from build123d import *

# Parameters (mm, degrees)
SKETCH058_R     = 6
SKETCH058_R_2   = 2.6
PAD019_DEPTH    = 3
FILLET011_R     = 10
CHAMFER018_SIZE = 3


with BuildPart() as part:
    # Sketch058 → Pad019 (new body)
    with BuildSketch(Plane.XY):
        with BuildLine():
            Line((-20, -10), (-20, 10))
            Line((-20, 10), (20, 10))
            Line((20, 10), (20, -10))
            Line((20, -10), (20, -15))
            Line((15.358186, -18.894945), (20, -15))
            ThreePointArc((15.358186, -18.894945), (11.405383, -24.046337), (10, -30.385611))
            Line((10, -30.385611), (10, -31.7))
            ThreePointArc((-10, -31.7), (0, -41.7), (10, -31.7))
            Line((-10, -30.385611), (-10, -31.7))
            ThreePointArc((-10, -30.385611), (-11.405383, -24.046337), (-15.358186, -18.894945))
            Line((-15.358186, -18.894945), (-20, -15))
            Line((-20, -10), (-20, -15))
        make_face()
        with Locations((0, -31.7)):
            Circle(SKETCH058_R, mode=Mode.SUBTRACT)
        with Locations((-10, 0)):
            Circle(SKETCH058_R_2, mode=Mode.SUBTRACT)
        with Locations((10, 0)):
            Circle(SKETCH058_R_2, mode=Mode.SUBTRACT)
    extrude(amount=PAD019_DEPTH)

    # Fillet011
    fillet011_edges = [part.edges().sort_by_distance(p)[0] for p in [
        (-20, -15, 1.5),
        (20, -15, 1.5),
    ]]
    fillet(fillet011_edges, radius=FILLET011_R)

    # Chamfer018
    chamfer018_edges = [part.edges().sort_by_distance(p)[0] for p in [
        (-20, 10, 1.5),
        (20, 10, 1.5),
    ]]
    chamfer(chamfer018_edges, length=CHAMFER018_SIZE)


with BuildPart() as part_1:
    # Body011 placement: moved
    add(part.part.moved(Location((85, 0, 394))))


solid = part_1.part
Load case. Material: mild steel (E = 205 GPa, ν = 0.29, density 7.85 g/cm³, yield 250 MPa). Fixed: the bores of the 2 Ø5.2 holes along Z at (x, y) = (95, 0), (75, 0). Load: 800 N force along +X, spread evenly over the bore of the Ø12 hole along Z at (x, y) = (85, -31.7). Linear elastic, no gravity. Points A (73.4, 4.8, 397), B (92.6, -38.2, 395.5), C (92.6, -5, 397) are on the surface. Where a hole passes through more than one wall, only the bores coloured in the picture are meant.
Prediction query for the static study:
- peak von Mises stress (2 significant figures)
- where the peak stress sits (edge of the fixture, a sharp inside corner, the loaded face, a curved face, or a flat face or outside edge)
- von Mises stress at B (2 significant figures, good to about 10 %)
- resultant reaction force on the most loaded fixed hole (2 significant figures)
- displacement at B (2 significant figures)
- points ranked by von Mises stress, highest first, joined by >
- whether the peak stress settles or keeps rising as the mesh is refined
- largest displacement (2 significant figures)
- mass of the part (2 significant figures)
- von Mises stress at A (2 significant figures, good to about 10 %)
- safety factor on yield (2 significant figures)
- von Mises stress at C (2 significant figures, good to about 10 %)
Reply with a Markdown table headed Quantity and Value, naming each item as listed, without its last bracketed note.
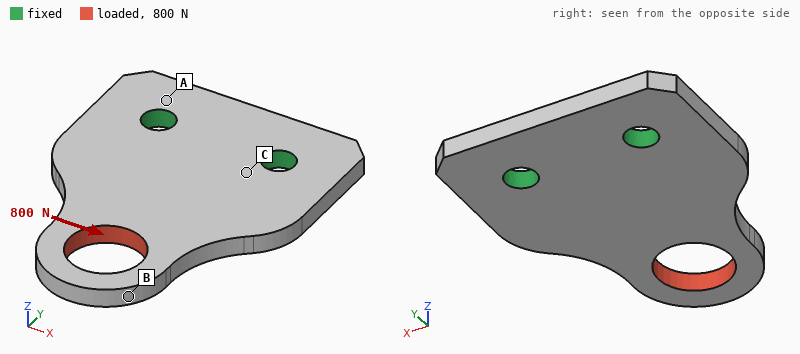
| Quantity | Value |
|---|---|
| peak von Mises stress | 96 MPa |
| where the peak stress sits | the loaded face |
| von Mises stress at B | 44 MPa |
| resultant reaction force on the most loaded fixed hole | 1.1 kN |
| displacement at B | 18 µm |
| points ranked by von Mises stress, highest first, joined by > | B > C > A |
| whether the peak stress settles or keeps rising as the mesh is refined | settles |
| largest displacement | 19 µm |
| mass of the part | 33 g |
| von Mises stress at A | 11 MPa |
| safety factor on yield | 2.6 |
| von Mises stress at C | 30 MPa |
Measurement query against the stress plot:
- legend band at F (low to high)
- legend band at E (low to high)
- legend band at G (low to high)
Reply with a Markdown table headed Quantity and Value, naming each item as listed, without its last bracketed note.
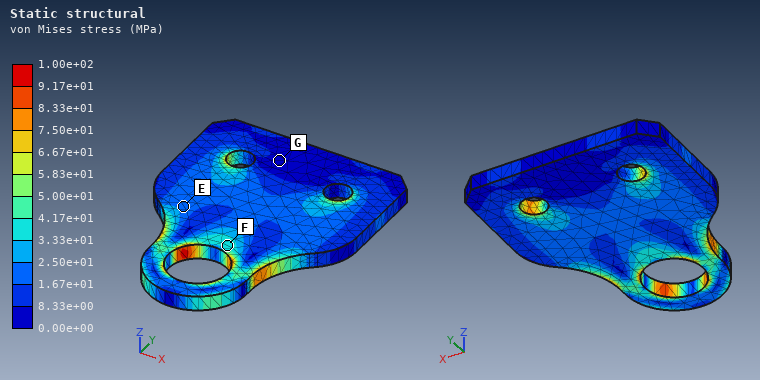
| Quantity | Value |
|---|---|
| legend band at F | 3.33e+01 to 4.17e+01 MPa |
| legend band at E | 1.67e+01 to 2.50e+01 MPa |
| legend band at G | 0.00e+00 to 8.33e+00 MPa |
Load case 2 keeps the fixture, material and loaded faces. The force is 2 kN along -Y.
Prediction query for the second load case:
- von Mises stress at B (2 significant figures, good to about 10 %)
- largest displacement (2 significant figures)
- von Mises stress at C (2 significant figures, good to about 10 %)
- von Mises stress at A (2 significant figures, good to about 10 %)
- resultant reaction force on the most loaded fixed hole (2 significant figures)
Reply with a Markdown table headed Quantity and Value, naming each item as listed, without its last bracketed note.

| Quantity | Value |
|---|---|
| von Mises stress at B | 11 MPa |
| largest displacement | 8.8 µm |
| von Mises stress at C | 28 MPa |
| von Mises stress at A | 6.7 MPa |
| resultant reaction force on the most loaded fixed hole | 1.0 kN |
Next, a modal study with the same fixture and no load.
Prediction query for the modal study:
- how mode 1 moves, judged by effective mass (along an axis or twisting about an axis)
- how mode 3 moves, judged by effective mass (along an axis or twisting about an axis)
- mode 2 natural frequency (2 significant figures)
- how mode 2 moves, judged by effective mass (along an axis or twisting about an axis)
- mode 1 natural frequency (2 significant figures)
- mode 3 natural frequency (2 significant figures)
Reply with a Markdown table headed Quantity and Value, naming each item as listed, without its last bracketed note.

| Quantity | Value |
|---|---|
| how mode 1 moves, judged by effective mass | along Z |
| how mode 3 moves, judged by effective mass | along Z |
| mode 2 natural frequency | 7700 Hz |
| how mode 2 moves, judged by effective mass | twisting about Y |
| mode 1 natural frequency | 2500 Hz |
| mode 3 natural frequency | 9100 Hz |
